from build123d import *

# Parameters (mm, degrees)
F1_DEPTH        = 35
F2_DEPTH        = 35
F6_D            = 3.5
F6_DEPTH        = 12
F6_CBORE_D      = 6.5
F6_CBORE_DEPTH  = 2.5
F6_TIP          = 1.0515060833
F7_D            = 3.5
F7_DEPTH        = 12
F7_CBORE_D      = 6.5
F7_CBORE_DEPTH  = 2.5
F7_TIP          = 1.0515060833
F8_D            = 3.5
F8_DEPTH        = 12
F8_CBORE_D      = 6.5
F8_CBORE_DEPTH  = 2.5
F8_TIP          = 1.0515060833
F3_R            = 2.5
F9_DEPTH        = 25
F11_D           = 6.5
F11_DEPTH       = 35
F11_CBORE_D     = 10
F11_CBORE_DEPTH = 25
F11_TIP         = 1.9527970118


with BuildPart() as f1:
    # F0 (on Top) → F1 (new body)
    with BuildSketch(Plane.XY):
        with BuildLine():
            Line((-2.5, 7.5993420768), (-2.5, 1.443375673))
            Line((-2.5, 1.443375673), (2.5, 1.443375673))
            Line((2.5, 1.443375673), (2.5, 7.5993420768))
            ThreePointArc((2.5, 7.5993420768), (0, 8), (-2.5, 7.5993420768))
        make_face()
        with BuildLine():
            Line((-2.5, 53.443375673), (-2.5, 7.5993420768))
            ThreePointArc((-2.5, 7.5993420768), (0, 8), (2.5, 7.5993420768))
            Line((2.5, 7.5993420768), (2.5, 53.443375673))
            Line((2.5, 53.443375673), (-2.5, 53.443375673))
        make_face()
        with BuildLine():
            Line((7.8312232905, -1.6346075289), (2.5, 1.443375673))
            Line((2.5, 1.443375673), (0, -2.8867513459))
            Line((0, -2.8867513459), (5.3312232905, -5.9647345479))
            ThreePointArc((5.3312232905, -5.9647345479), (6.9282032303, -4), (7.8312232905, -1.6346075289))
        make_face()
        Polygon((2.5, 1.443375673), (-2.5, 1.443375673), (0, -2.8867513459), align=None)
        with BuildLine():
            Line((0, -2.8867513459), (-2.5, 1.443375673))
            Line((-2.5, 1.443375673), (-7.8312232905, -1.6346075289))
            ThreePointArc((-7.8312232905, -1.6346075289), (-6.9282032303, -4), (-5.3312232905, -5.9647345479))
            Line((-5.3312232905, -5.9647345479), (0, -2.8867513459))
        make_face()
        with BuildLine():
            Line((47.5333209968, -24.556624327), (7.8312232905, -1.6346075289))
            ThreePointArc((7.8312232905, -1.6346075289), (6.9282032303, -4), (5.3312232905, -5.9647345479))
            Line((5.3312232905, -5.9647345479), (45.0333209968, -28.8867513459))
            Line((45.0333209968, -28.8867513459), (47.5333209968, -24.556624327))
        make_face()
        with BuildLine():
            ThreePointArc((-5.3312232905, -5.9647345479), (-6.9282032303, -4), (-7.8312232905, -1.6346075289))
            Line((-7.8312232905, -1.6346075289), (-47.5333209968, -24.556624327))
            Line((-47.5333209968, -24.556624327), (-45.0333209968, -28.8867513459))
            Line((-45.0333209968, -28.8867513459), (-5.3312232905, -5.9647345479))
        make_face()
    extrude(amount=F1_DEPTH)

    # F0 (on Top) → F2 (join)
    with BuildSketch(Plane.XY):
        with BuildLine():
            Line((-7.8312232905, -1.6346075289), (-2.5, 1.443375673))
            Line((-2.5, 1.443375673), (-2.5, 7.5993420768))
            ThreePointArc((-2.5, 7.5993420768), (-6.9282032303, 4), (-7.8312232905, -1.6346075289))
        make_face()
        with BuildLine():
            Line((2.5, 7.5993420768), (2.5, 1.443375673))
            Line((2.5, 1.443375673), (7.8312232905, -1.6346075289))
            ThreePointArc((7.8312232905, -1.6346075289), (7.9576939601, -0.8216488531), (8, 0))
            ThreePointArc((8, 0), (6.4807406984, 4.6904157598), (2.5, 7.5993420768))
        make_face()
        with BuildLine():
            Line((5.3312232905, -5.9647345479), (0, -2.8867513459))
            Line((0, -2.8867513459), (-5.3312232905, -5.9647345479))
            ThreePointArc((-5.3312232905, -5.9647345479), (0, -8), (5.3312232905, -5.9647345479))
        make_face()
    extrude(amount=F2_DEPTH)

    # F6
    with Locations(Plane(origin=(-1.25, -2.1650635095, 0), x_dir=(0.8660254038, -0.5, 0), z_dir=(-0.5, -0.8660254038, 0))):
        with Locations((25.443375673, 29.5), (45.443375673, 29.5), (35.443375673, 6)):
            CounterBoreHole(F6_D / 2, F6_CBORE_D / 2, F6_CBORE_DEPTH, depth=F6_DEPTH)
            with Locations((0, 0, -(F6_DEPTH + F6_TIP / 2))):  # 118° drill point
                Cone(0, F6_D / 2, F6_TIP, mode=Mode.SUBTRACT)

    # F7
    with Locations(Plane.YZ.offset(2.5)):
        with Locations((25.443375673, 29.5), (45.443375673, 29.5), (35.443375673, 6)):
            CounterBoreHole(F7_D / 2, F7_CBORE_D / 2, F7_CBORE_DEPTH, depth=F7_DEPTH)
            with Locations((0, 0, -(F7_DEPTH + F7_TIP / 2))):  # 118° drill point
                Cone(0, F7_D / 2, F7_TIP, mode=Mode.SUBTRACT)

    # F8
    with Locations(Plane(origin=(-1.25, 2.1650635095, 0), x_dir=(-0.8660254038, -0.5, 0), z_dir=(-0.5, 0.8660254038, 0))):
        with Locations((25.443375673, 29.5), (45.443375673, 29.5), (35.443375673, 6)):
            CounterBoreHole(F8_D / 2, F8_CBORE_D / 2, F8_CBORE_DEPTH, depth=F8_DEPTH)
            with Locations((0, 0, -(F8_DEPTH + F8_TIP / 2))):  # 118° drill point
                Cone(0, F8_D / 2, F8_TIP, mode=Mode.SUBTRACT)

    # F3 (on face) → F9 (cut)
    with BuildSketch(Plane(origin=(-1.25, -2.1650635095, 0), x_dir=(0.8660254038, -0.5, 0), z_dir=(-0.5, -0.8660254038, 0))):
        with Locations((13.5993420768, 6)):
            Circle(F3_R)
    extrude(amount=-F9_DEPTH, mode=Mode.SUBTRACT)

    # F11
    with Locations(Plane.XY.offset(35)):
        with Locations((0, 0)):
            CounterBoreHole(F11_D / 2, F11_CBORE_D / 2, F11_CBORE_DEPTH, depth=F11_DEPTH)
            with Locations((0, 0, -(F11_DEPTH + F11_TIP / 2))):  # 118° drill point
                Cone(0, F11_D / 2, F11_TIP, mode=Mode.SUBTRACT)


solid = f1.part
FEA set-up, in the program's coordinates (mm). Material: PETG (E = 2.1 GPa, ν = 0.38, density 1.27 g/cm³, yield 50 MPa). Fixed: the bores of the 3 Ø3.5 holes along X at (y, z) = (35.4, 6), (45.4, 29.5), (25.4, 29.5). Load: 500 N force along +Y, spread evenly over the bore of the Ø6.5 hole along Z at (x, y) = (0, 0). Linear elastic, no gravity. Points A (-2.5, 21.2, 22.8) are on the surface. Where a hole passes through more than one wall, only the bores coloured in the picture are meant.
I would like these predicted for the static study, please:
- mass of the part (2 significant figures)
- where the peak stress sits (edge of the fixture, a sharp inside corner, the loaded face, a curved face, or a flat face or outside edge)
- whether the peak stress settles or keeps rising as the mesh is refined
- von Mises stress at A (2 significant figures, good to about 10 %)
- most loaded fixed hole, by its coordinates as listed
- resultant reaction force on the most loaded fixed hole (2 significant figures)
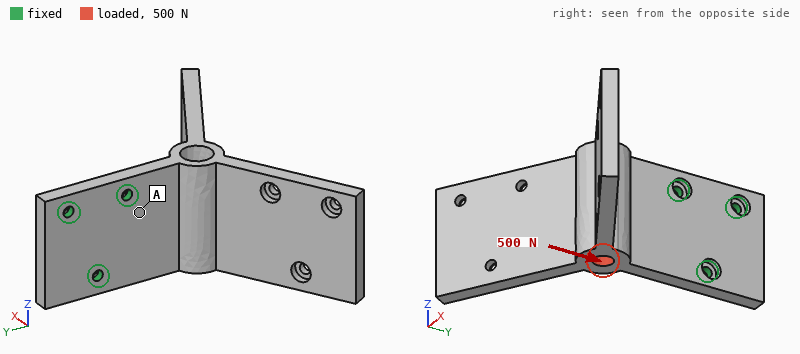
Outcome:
35 g
edge of the fixture
keeps rising
1.5 MPa
(35.4, 6)
440 N
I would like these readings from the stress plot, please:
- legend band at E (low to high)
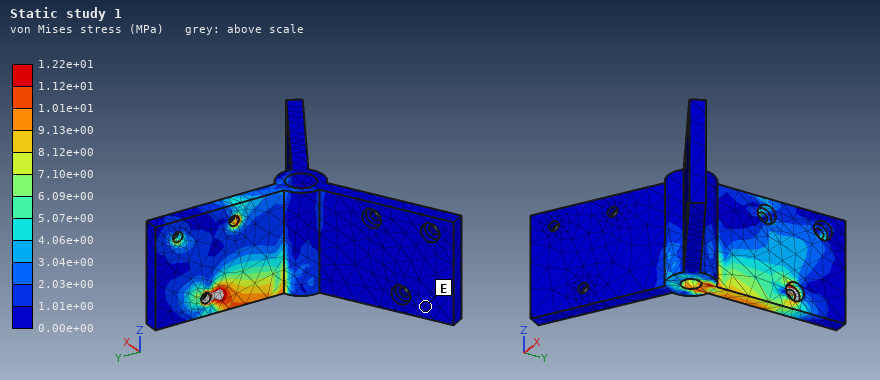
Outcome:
0.00e+00 to 1.01e+00 MPa
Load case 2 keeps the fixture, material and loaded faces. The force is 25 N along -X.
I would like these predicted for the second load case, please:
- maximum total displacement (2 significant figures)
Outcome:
1.4 mm
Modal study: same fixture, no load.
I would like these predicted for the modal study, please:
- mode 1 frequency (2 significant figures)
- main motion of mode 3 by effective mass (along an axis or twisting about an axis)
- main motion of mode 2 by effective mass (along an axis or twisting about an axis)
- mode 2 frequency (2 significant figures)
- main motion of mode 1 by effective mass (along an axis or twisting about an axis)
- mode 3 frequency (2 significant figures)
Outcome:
120 Hz
along Y
twisting about Y
310 Hz
along X
440 Hz
